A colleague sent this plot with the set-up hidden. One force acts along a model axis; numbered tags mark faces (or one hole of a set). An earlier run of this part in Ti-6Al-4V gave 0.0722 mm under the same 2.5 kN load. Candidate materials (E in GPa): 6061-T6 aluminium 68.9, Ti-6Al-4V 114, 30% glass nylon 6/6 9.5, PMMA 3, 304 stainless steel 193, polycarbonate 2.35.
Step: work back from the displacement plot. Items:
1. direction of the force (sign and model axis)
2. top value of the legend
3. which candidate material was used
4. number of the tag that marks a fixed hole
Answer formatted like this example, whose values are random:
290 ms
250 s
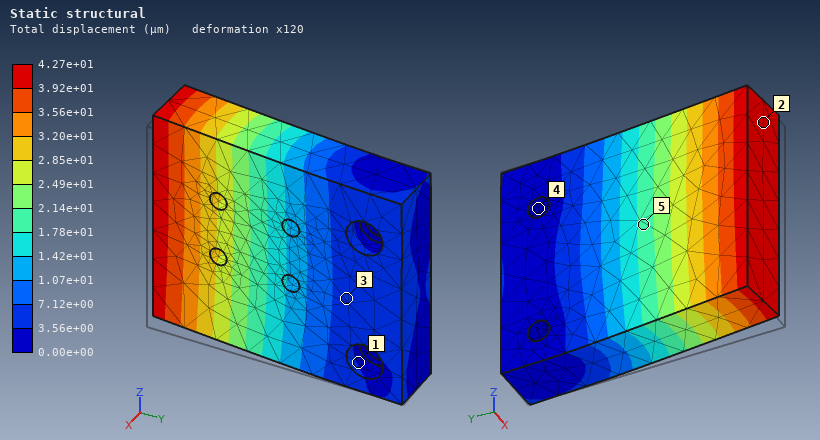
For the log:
-X
4.27e+01 µm
304 stainless steel
4
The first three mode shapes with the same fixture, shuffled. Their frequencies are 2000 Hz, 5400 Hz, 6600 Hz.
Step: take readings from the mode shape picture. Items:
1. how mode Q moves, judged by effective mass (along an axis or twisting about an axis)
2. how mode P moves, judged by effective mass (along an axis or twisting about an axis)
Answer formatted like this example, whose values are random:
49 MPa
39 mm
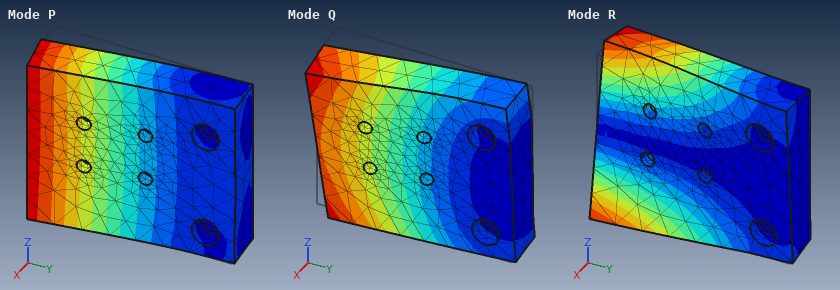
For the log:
along Z
along X
